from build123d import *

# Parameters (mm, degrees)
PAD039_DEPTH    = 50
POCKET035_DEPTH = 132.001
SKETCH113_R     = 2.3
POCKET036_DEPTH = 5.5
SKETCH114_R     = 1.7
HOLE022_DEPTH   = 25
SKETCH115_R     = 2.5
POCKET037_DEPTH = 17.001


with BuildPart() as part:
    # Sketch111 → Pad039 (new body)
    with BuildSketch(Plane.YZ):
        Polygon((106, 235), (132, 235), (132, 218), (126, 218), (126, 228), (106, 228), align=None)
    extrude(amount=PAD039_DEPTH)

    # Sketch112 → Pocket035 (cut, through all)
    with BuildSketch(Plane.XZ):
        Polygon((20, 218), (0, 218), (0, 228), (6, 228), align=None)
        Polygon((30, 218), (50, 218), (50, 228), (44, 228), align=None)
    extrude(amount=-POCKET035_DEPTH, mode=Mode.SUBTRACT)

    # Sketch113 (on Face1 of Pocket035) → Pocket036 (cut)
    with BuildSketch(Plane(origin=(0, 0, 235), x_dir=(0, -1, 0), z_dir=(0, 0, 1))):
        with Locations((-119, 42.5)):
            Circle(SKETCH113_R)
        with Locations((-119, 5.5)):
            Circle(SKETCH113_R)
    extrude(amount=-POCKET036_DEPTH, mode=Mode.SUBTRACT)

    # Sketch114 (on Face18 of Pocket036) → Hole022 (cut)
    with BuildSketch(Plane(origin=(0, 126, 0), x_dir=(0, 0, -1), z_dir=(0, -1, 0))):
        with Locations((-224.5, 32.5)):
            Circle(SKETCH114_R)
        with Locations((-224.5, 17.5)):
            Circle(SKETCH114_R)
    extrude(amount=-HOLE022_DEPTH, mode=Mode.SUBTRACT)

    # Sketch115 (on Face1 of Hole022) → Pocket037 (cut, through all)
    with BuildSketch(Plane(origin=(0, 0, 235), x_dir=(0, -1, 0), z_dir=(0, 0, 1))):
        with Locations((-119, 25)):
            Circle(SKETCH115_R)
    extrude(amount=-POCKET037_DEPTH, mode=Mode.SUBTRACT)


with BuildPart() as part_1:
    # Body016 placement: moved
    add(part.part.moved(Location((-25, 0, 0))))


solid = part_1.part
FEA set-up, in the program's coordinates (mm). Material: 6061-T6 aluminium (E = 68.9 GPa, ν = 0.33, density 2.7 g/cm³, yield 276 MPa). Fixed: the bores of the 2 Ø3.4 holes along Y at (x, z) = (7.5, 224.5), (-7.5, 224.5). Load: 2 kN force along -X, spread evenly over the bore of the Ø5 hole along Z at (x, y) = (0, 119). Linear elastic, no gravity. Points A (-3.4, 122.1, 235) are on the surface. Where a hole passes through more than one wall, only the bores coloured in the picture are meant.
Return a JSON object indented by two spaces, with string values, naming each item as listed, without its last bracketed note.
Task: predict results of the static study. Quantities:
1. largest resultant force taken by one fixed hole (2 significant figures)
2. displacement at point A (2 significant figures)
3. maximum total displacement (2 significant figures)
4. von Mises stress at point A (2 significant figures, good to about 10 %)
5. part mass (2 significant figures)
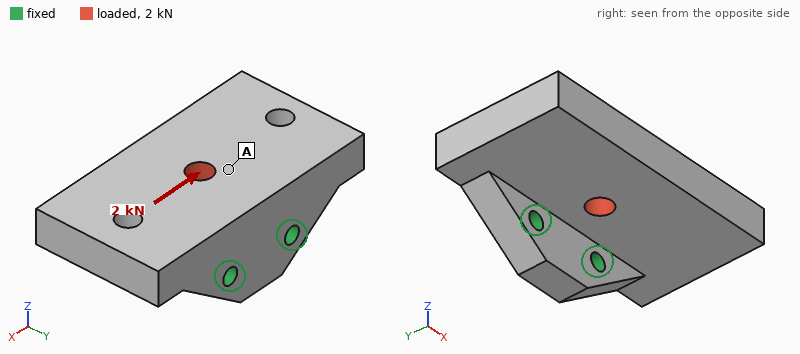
{
  "largest resultant force taken by one fixed hole": "1.6 kN",
  "displacement at point A": "10.0 µm",
  "maximum total displacement": "31 µm",
  "von Mises stress at point A": "15 MPa",
  "part mass": "27 g"
}
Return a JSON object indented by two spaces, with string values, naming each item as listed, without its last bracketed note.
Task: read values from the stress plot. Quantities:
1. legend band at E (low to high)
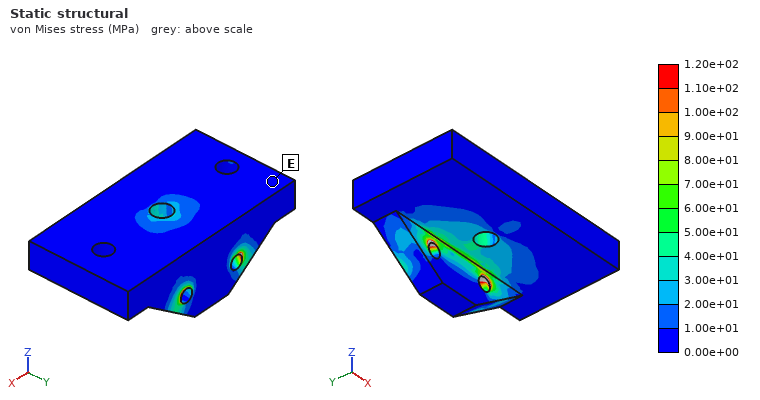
{
  "legend band at E": "0.00e+00 to 1.00e+01 MPa"
}
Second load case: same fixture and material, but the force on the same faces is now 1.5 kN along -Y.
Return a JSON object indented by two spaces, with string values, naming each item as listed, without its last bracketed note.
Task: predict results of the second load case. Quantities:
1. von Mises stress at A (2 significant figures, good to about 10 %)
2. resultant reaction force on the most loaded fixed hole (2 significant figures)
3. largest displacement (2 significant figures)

{
  "von Mises stress at A": "13 MPa",
  "resultant reaction force on the most loaded fixed hole": "750 N",
  "largest displacement": "32 µm"
}
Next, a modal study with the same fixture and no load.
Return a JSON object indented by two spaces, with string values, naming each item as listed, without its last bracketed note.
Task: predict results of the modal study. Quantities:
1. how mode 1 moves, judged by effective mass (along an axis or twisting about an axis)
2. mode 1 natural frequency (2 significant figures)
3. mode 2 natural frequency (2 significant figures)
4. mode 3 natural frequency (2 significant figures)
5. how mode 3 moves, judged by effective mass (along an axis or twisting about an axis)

{
  "how mode 1 moves, judged by effective mass": "along Z",
  "mode 1 natural frequency": "5100 Hz",
  "mode 2 natural frequency": "7400 Hz",
  "mode 3 natural frequency": "9700 Hz",
  "how mode 3 moves, judged by effective mass": "along X"
}
